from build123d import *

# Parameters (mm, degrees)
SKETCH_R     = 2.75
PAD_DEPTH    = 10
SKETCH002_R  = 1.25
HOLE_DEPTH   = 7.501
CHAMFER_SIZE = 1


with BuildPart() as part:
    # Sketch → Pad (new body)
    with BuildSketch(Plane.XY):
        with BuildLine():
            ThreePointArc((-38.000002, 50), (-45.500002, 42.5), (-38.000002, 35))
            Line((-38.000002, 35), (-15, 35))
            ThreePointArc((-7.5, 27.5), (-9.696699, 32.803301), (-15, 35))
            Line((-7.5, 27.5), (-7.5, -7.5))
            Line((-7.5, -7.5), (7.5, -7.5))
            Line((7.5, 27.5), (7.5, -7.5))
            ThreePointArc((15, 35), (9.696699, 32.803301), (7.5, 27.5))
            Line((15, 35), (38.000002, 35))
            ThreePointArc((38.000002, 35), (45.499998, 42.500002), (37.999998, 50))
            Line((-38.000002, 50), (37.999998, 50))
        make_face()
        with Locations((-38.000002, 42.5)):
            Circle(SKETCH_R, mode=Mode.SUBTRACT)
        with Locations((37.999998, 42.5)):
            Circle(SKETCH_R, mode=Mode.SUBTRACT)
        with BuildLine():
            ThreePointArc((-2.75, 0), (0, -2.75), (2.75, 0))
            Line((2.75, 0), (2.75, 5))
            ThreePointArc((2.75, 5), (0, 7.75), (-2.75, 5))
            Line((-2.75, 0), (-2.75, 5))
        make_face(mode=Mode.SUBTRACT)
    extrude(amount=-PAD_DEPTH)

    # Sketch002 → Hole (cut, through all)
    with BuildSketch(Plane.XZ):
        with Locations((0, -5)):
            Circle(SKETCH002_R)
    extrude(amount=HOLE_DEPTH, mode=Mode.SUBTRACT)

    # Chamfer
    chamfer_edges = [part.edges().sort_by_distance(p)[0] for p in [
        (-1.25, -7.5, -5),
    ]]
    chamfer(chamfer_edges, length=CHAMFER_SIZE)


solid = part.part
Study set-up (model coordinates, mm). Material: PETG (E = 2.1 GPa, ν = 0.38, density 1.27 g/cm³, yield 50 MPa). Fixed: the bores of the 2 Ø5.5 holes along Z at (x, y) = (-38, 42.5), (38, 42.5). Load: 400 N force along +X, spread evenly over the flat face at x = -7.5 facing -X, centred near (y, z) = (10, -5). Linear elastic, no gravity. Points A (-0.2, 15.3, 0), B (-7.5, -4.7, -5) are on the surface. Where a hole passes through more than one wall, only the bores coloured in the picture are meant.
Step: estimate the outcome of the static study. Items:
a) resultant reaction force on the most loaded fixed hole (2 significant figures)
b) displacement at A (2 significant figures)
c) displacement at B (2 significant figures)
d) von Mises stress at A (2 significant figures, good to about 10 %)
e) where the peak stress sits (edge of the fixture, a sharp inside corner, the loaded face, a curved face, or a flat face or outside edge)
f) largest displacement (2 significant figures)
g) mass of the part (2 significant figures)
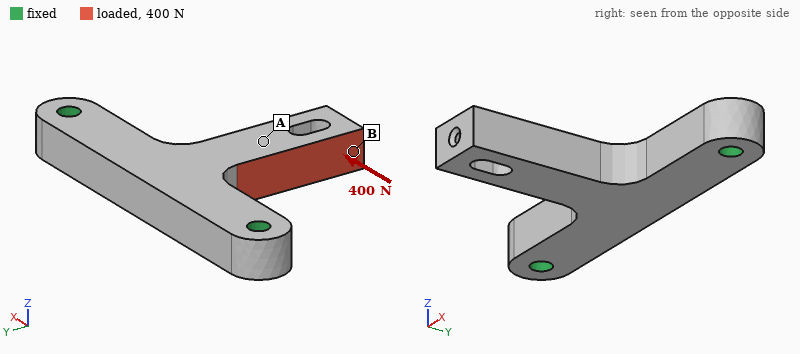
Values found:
300 N
0.49 mm
1.2 mm
5.3 MPa
a curved face
1.3 mm
24 g
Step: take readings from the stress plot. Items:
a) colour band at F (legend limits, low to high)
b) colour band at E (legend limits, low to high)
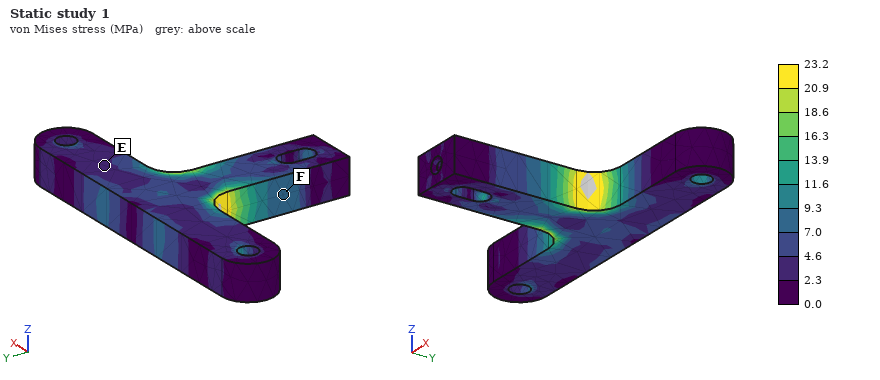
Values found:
7.0 to 9.3 MPa
2.3 to 4.6 MPa
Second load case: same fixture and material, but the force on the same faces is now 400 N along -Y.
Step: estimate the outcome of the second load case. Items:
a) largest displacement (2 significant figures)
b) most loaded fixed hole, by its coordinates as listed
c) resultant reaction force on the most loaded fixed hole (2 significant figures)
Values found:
0.57 mm
(-38, 42.5)
260 N
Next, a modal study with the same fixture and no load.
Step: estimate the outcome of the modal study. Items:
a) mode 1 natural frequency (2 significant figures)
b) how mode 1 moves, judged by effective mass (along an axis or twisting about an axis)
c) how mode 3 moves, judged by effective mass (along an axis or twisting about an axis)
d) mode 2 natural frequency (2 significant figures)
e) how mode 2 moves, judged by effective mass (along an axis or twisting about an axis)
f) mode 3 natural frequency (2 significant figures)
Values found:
590 Hz
along Z
along Y
1400 Hz
along X
1900 Hz
